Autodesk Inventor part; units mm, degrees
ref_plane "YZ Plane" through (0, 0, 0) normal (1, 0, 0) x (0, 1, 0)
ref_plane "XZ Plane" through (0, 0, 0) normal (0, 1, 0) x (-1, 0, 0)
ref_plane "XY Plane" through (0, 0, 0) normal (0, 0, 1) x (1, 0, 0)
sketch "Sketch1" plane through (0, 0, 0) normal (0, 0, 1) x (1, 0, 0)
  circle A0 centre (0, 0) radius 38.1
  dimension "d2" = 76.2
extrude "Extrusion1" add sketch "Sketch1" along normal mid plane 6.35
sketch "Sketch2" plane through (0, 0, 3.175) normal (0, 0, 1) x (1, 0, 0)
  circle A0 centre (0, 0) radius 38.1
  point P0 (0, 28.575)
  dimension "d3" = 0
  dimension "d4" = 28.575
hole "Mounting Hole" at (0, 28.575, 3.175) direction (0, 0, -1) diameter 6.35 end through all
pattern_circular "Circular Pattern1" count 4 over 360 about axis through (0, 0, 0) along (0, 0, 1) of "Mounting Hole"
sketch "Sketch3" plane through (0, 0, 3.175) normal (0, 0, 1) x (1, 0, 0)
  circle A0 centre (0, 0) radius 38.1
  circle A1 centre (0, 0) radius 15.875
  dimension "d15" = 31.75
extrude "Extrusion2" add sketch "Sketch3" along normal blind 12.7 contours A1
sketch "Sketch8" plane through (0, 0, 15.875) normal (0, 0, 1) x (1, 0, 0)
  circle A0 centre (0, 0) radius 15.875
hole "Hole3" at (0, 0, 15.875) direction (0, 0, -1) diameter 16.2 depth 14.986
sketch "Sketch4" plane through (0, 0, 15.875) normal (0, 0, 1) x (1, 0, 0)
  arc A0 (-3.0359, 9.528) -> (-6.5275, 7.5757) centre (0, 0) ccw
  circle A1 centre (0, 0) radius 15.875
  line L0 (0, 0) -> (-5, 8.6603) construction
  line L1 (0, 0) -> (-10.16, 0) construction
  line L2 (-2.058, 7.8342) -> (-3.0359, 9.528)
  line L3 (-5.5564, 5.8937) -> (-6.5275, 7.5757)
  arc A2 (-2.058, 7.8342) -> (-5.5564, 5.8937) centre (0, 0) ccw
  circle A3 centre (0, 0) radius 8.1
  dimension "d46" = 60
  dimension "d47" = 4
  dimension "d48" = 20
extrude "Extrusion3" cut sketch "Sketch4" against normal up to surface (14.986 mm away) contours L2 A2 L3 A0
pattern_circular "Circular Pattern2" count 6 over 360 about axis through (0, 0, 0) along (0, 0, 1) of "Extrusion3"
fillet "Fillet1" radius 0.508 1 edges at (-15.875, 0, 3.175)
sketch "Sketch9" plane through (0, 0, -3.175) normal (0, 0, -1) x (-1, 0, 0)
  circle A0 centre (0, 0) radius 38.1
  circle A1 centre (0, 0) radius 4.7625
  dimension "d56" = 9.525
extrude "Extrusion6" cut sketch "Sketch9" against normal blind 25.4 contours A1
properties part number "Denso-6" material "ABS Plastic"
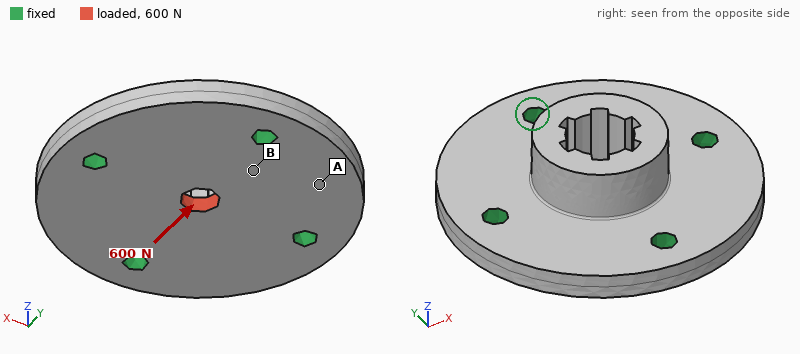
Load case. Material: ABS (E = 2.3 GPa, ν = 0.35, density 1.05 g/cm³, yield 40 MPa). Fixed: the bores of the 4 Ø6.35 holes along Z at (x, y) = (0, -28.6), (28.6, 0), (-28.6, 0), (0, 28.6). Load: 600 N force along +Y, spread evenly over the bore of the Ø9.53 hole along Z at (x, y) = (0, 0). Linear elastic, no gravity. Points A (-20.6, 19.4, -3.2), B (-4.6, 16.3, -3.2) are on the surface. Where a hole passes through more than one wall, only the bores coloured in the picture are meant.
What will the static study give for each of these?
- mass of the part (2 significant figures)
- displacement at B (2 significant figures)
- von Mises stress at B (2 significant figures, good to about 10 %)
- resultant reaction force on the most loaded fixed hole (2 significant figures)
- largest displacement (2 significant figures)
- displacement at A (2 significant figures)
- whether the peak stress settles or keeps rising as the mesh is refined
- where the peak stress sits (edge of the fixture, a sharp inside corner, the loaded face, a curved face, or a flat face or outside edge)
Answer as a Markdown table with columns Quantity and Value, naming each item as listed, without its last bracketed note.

| Quantity | Value |
|---|---|
| mass of the part | 36 g |
| displacement at B | 10 µm |
| von Mises stress at B | 2.3 MPa |
| resultant reaction force on the most loaded fixed hole | 200 N |
| largest displacement | 31 µm |
| displacement at A | 7.6 µm |
| whether the peak stress settles or keeps rising as the mesh is refined | keeps rising |
| where the peak stress sits | a sharp inside corner |
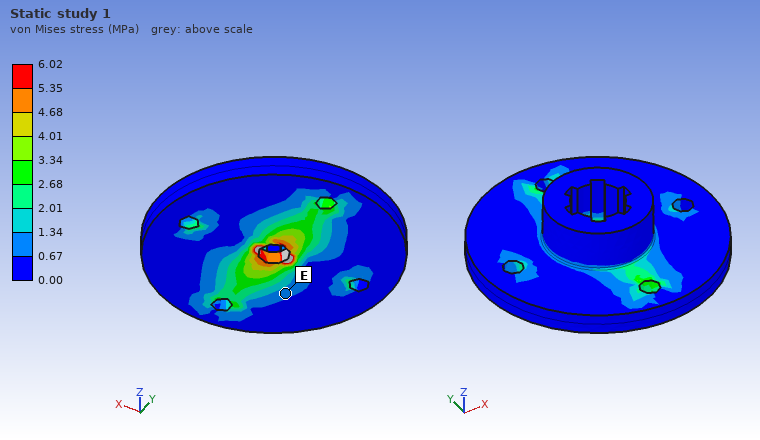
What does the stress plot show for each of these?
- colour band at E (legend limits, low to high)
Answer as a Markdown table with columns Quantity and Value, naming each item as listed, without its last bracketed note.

| Quantity | Value |
|---|---|
| colour band at E | 0.67 to 1.34 MPa |
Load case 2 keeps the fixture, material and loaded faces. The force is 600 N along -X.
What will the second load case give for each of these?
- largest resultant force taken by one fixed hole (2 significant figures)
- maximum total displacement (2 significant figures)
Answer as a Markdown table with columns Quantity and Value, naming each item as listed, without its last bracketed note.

| Quantity | Value |
|---|---|
| largest resultant force taken by one fixed hole | 200 N |
| maximum total displacement | 31 µm |
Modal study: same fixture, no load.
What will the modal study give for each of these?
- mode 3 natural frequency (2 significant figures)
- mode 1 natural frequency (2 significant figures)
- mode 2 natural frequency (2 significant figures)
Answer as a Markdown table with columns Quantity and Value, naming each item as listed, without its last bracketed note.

| Quantity | Value |
|---|---|
| mode 3 natural frequency | 4100 Hz |
| mode 1 natural frequency | 4100 Hz |
| mode 2 natural frequency | 4100 Hz |
